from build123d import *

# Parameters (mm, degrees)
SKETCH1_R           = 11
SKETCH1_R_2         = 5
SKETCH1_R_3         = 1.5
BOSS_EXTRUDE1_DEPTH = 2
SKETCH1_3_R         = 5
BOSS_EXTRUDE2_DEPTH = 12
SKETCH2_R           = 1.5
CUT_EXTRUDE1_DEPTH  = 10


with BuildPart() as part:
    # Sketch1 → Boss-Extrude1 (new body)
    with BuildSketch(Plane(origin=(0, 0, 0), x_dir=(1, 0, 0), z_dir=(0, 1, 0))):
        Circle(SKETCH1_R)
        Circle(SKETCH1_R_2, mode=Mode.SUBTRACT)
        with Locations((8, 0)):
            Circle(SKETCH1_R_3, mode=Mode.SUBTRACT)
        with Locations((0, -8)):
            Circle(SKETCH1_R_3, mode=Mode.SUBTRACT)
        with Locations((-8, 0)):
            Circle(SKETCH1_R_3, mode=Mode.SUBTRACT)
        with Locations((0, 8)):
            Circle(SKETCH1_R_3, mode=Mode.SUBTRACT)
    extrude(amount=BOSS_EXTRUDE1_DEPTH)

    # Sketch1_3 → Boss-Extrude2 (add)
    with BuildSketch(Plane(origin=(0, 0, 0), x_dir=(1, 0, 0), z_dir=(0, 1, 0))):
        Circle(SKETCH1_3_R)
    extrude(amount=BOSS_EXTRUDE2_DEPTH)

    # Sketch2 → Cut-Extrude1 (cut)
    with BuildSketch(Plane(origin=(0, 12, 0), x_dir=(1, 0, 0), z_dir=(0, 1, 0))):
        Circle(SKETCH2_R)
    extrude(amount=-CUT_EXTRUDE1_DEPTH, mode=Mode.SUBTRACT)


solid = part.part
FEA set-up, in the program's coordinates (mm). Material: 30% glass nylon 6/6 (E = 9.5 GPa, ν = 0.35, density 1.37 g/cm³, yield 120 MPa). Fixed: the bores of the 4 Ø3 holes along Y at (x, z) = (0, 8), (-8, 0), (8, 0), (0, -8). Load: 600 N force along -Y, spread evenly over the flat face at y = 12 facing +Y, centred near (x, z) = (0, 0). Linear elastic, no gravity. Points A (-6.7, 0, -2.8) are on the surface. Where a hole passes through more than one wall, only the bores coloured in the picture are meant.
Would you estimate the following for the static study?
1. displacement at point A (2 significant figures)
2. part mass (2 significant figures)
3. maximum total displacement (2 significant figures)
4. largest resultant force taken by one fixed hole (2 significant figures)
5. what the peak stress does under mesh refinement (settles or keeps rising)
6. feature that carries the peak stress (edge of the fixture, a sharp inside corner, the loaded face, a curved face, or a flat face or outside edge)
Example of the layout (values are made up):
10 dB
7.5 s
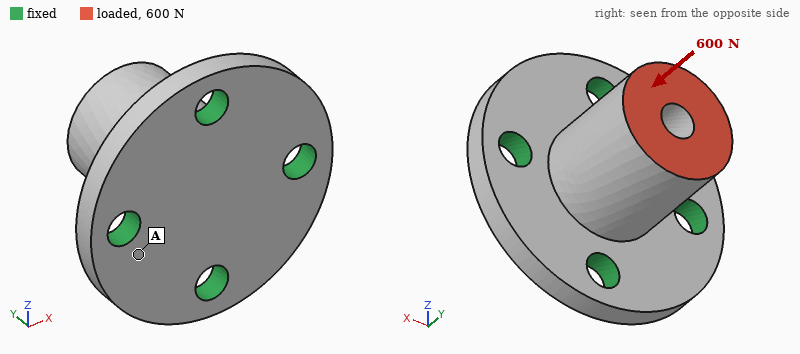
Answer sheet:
6.1 µm
1.9 g
27 µm
160 N
keeps rising
edge of the fixture
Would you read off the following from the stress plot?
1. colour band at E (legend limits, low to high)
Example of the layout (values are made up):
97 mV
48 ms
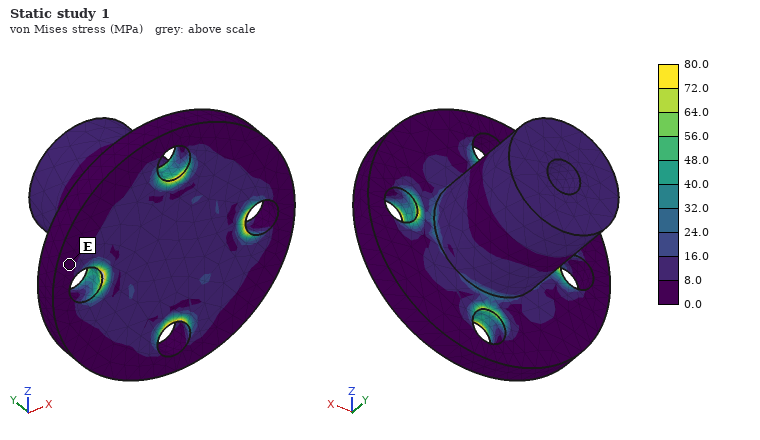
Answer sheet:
0.0 to 8.0 MPa
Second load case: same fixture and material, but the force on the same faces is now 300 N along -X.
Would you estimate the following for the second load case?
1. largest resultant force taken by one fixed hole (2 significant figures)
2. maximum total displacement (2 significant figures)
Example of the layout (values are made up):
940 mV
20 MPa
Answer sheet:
270 N
0.10 mm
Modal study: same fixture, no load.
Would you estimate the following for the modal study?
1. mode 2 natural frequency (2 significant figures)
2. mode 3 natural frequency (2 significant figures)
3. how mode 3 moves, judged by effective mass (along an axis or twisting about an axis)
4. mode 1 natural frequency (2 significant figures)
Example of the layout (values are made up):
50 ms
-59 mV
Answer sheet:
15 kHz
24 kHz
along Y
15 kHz
